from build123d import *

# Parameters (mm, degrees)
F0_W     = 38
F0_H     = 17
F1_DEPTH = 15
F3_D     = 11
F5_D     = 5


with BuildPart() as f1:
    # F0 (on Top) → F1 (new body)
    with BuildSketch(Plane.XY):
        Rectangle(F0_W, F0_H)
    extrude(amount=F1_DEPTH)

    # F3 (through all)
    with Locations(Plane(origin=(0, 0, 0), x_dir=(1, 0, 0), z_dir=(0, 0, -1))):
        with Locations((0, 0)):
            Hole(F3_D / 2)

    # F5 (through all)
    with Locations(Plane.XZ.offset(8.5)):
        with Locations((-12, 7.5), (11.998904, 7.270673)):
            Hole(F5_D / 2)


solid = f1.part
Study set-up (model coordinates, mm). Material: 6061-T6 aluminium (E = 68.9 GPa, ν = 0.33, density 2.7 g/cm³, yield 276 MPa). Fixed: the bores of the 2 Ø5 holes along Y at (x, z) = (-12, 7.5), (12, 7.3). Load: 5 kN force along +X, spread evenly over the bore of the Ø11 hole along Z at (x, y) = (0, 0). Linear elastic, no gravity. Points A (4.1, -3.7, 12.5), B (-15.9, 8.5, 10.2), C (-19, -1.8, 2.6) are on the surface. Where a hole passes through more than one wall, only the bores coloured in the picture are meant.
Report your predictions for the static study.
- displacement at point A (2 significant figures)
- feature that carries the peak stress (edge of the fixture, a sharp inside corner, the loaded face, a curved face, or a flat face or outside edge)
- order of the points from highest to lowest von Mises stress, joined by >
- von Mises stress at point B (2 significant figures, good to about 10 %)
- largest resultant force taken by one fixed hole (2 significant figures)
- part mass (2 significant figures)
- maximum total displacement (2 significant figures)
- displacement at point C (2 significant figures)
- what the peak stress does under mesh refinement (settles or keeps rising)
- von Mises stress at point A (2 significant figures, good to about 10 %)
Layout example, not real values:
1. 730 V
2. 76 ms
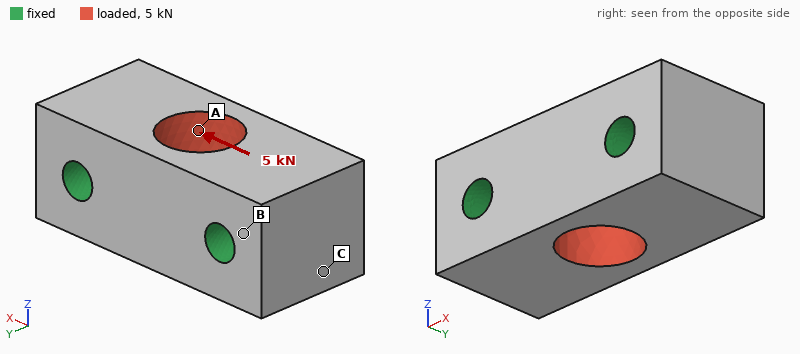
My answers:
1. 1.6 µm
2. edge of the fixture
3. A > B > C
4. 4.4 MPa
5. 2.5 kN
6. 21 g
7. 1.9 µm
8. 0.45 µm
9. keeps rising
10. 15 MPa
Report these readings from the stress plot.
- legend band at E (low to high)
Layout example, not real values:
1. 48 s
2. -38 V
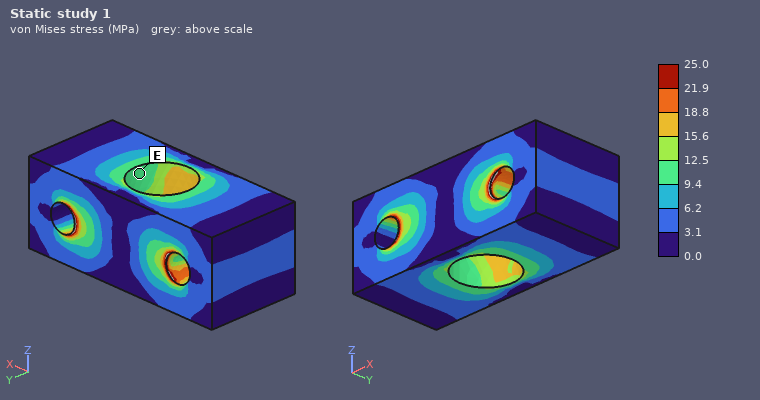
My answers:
1. 9.4 to 12.5 MPa
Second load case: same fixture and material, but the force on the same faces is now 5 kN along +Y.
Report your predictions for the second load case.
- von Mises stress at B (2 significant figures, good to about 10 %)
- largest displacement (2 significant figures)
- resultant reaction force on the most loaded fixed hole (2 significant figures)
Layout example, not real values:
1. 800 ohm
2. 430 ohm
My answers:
1. 5.6 MPa
2. 6.6 µm
3. 2.5 kN
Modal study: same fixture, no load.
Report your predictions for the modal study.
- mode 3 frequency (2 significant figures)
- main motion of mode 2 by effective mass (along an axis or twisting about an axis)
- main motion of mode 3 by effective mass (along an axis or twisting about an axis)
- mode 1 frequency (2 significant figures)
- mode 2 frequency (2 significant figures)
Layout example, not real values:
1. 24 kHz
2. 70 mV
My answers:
1. 70 kHz
2. twisting about X
3. along Y
4. 55 kHz
5. 66 kHz
